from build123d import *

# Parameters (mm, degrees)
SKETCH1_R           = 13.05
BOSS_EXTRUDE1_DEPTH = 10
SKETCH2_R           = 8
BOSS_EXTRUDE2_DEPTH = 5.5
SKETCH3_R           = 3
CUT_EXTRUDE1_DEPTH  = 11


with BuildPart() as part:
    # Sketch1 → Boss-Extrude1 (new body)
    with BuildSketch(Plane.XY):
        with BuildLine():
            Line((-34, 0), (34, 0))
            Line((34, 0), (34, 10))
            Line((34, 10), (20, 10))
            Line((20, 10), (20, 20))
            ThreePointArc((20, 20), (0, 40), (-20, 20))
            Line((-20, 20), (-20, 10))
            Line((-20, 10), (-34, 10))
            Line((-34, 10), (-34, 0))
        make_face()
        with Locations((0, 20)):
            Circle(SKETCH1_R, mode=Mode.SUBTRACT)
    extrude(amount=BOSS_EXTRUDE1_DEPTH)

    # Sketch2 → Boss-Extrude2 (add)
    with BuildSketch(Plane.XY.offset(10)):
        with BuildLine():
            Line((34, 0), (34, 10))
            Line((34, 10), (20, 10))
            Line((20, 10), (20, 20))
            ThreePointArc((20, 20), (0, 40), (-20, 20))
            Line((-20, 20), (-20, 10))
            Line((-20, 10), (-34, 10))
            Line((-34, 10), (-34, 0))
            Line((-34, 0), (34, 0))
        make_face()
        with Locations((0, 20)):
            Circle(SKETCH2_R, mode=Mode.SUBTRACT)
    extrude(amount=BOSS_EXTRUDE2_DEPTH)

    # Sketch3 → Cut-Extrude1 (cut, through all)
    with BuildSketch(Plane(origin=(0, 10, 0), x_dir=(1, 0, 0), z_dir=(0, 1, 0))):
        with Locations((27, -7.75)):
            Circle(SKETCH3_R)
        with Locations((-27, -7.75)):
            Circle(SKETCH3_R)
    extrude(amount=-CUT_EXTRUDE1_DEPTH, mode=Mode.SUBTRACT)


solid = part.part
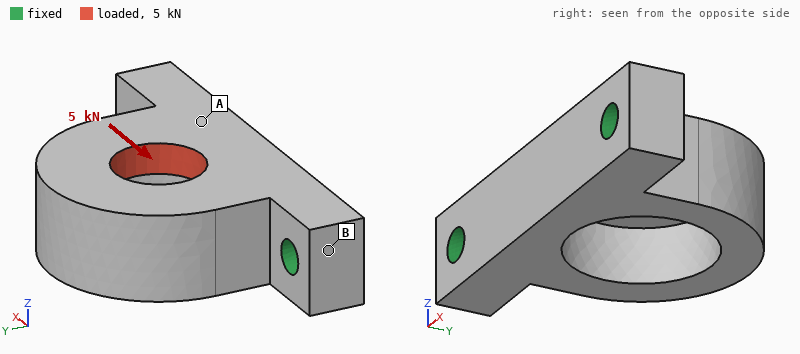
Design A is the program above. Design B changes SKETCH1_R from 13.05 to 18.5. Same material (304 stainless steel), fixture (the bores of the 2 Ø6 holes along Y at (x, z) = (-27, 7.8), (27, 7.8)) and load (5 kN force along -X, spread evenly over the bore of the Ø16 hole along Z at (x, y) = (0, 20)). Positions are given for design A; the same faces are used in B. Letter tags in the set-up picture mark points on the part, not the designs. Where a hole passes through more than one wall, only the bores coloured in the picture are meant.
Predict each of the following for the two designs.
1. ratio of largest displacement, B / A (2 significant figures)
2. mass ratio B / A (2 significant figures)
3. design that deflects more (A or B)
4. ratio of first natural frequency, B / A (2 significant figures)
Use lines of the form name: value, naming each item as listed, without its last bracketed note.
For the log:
ratio of largest displacement, B / A: 2.2
mass ratio B / A: 0.72
design that deflects more: B
ratio of first natural frequency, B / A: 0.97
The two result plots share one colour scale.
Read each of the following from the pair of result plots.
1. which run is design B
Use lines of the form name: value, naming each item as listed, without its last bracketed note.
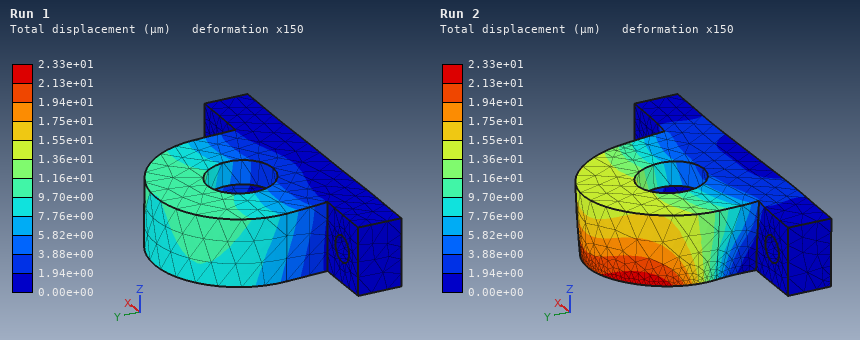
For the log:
which run is design B: Run 2
